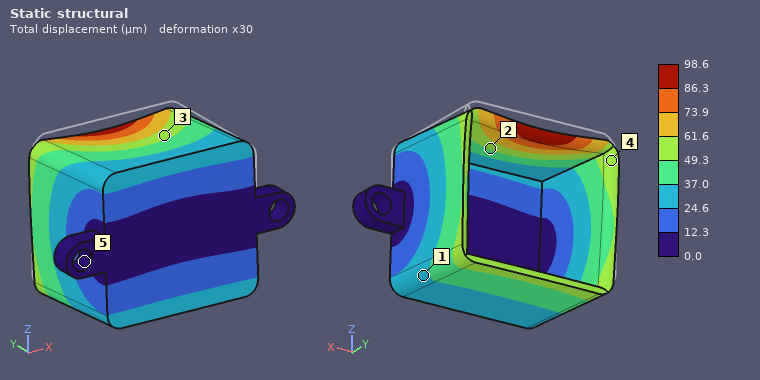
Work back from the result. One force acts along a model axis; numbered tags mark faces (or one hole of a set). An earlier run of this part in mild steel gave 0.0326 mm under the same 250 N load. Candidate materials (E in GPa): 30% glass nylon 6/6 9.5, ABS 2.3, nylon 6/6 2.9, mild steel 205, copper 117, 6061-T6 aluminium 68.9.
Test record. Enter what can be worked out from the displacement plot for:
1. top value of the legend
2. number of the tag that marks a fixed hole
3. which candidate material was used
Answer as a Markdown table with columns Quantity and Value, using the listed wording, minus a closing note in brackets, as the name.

| Quantity | Value |
|---|---|
| top value of the legend | 98.6 µm |
| number of the tag that marks a fixed hole | 5 |
| which candidate material was used | 6061-T6 aluminium |
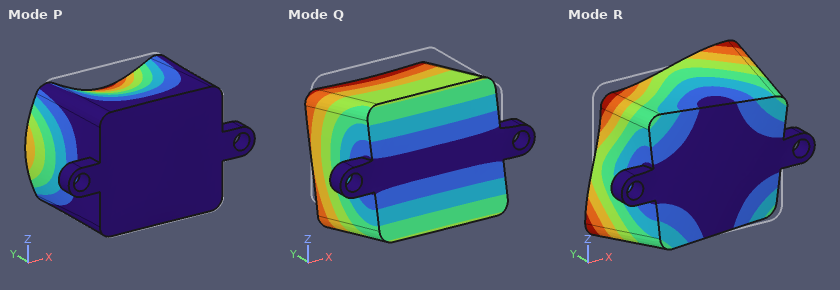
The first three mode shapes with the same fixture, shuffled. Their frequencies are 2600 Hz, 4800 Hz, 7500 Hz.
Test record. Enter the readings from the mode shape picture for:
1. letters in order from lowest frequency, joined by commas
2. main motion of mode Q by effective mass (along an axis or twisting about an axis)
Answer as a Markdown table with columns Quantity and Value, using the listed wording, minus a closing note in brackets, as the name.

| Quantity | Value |
|---|---|
| letters in order from lowest frequency, joined by commas | Q, R, P |
| main motion of mode Q by effective mass | along Z |
